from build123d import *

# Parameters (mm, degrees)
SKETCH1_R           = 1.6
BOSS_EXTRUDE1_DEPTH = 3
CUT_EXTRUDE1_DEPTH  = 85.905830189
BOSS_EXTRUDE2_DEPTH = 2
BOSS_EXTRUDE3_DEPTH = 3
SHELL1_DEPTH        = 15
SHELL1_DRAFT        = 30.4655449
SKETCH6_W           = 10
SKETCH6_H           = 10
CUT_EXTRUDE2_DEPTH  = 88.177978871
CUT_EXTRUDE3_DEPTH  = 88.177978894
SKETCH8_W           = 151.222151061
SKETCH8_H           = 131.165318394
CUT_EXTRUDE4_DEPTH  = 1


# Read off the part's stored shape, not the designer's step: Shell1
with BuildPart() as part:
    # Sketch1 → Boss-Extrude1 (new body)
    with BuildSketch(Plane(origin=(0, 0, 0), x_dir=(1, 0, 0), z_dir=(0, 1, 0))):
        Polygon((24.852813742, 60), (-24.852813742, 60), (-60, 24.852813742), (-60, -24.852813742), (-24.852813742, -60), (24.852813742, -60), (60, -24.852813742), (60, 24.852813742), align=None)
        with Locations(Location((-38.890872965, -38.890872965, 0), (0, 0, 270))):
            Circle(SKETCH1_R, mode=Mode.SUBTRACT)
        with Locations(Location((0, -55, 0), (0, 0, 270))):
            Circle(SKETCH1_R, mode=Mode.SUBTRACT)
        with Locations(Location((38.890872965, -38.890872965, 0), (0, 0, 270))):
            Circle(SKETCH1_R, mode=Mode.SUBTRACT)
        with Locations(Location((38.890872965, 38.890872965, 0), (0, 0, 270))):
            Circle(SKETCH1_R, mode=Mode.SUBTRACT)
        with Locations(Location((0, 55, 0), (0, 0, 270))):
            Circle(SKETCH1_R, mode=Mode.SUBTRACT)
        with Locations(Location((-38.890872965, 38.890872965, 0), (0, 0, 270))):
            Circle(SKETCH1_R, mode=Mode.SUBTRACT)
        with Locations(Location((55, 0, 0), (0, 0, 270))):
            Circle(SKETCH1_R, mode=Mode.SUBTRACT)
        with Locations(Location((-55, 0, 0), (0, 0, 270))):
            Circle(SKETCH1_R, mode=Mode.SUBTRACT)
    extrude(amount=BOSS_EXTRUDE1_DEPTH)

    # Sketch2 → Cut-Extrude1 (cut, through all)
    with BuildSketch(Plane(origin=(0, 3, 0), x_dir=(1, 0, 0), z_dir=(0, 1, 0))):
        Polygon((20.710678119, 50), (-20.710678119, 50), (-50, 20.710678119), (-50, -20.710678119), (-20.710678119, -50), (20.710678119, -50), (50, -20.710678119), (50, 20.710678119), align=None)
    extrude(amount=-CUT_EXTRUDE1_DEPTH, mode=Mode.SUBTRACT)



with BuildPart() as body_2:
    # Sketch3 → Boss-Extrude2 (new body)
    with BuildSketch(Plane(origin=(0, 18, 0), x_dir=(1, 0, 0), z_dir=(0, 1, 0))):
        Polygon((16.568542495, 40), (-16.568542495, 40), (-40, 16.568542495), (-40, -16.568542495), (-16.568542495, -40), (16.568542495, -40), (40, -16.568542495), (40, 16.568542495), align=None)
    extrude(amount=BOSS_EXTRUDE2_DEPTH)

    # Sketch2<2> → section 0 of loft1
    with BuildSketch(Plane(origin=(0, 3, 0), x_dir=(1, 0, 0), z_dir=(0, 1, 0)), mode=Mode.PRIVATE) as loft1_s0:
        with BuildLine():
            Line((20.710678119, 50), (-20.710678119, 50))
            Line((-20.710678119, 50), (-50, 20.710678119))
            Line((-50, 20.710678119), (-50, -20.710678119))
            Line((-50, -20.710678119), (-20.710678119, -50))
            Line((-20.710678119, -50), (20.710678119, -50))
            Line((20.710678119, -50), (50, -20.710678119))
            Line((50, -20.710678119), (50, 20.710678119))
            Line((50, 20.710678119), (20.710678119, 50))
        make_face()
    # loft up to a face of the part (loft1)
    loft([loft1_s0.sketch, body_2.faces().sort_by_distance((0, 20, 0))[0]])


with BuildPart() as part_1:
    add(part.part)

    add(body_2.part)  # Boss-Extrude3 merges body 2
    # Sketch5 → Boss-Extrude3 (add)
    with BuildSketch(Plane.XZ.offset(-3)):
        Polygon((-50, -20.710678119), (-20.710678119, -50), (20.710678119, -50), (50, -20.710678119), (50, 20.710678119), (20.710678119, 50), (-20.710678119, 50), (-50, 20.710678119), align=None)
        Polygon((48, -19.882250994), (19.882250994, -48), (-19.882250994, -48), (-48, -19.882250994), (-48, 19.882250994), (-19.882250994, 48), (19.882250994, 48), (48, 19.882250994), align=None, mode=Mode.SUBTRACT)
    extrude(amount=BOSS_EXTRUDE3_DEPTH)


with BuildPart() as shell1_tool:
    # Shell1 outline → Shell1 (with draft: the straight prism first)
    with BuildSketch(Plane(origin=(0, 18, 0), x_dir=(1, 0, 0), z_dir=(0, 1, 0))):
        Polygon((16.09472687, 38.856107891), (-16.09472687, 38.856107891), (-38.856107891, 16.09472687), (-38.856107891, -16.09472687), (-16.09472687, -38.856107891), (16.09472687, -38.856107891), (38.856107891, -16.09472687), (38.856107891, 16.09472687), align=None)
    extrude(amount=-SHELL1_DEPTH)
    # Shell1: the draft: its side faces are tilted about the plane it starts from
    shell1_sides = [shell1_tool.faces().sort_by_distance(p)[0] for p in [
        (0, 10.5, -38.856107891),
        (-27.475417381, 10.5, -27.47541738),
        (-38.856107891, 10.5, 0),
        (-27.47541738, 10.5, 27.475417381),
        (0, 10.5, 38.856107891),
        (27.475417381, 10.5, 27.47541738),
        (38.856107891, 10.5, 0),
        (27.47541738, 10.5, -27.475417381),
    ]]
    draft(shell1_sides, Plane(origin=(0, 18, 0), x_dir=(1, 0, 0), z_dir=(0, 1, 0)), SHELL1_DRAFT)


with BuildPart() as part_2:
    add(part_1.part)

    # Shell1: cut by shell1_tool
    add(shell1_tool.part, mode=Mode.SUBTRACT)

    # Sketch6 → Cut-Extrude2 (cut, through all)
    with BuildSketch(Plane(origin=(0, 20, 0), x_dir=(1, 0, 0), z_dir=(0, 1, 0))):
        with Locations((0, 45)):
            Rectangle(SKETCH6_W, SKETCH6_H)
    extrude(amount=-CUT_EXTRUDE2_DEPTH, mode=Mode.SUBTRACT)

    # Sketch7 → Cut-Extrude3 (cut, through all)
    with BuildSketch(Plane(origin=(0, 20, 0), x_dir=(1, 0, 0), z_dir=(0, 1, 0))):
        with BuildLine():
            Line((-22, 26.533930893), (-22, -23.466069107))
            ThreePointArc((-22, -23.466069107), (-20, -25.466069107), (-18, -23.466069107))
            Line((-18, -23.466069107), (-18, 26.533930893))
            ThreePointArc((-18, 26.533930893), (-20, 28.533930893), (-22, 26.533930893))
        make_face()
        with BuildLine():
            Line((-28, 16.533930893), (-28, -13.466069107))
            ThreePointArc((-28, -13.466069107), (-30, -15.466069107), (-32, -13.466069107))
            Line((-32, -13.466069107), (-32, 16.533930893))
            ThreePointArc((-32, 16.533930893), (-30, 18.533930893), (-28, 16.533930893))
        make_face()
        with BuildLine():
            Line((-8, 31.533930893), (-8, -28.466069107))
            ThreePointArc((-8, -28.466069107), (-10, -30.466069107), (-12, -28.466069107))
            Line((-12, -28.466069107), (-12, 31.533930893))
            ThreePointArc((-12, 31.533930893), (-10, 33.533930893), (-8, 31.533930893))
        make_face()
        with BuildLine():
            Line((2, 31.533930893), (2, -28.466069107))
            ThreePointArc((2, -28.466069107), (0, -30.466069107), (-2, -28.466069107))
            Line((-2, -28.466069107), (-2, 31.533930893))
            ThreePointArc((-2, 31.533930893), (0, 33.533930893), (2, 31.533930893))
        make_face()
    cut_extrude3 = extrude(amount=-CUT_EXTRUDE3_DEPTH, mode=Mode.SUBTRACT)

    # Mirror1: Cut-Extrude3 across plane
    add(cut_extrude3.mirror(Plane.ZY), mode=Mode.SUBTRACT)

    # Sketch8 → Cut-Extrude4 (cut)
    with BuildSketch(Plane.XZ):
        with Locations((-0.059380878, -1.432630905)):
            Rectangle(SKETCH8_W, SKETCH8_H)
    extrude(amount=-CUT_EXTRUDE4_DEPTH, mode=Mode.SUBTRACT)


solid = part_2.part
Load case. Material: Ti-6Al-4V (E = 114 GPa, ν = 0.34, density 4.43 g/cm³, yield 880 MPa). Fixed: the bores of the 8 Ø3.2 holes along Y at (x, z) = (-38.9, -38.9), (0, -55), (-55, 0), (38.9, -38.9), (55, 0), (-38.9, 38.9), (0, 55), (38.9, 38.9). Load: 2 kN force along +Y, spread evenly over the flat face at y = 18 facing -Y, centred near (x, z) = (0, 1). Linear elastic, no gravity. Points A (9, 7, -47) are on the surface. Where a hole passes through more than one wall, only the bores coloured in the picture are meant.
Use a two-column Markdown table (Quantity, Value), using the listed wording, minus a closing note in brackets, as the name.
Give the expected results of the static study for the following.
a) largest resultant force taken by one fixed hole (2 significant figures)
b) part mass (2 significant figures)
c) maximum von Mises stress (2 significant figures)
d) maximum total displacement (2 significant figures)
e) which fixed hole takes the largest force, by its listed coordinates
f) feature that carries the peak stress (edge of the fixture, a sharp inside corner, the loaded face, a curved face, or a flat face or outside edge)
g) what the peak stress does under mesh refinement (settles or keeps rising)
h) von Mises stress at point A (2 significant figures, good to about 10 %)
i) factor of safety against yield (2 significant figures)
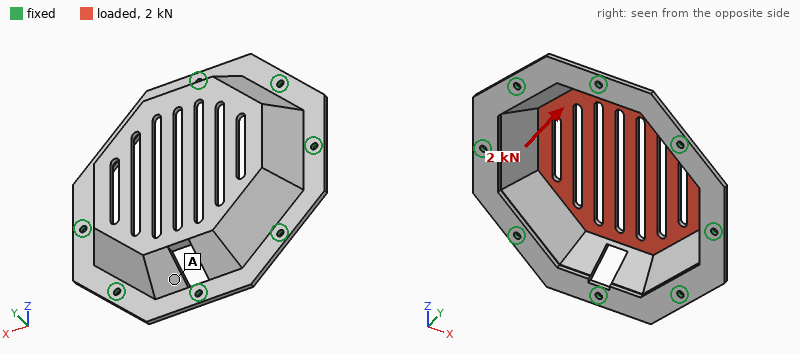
| Quantity | Value |
|---|---|
| largest resultant force taken by one fixed hole | 530 N |
| part mass | 120 g |
| maximum von Mises stress | 310 MPa |
| maximum total displacement | 0.75 mm |
| which fixed hole takes the largest force, by its listed coordinates | (0, 55) |
| feature that carries the peak stress | the loaded face |
| what the peak stress does under mesh refinement | settles |
| von Mises stress at point A | 41 MPa |
| factor of safety against yield | 2.9 |
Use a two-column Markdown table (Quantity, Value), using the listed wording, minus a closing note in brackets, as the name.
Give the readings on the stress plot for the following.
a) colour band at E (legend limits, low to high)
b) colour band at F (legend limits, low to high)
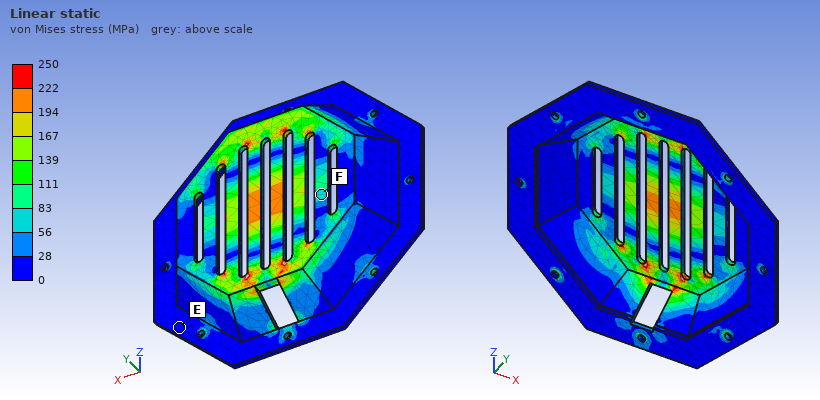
| Quantity | Value |
|---|---|
| colour band at E | 0 to 28 MPa |
| colour band at F | 56 to 83 MPa |
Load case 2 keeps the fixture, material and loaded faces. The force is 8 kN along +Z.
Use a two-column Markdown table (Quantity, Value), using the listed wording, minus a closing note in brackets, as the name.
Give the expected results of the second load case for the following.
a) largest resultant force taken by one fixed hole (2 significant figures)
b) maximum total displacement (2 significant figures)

| Quantity | Value |
|---|---|
| largest resultant force taken by one fixed hole | 1.3 kN |
| maximum total displacement | 0.11 mm |
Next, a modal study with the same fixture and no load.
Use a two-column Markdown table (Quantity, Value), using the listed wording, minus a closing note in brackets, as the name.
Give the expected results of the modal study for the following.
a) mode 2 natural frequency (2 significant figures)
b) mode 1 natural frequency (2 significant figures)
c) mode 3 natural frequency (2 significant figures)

| Quantity | Value |
|---|---|
| mode 2 natural frequency | 2100 Hz |
| mode 1 natural frequency | 1800 Hz |
| mode 3 natural frequency | 2400 Hz |
